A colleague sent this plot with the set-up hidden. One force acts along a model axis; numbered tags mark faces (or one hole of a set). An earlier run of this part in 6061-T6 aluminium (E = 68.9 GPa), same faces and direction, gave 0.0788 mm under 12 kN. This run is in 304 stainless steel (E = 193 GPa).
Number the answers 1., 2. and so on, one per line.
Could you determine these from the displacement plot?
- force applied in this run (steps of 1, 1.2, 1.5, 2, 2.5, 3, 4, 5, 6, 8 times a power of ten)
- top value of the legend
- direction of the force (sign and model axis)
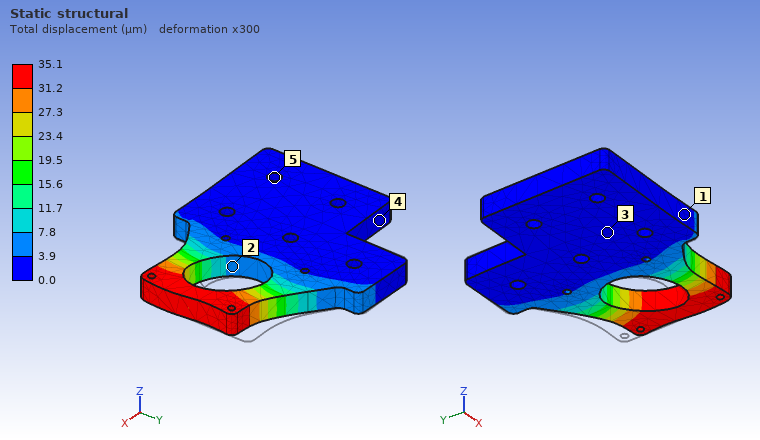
1. 15 kN
2. 35.1 µm
3. -Y
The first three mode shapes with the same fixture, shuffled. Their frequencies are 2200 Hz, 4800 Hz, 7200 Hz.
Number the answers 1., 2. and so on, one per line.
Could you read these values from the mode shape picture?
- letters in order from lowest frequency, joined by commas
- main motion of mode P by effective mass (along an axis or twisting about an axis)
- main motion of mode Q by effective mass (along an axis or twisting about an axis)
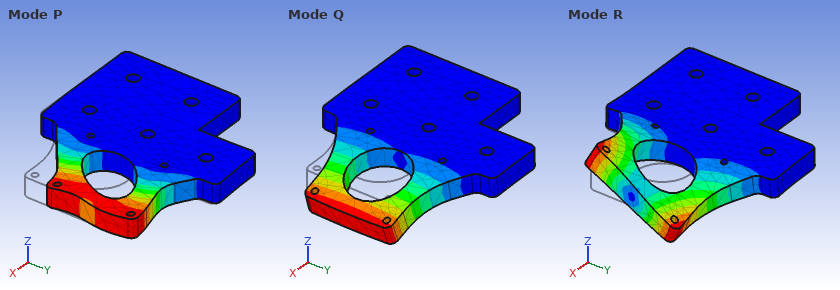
1. Q, R, P
2. along Y
3. along Z
